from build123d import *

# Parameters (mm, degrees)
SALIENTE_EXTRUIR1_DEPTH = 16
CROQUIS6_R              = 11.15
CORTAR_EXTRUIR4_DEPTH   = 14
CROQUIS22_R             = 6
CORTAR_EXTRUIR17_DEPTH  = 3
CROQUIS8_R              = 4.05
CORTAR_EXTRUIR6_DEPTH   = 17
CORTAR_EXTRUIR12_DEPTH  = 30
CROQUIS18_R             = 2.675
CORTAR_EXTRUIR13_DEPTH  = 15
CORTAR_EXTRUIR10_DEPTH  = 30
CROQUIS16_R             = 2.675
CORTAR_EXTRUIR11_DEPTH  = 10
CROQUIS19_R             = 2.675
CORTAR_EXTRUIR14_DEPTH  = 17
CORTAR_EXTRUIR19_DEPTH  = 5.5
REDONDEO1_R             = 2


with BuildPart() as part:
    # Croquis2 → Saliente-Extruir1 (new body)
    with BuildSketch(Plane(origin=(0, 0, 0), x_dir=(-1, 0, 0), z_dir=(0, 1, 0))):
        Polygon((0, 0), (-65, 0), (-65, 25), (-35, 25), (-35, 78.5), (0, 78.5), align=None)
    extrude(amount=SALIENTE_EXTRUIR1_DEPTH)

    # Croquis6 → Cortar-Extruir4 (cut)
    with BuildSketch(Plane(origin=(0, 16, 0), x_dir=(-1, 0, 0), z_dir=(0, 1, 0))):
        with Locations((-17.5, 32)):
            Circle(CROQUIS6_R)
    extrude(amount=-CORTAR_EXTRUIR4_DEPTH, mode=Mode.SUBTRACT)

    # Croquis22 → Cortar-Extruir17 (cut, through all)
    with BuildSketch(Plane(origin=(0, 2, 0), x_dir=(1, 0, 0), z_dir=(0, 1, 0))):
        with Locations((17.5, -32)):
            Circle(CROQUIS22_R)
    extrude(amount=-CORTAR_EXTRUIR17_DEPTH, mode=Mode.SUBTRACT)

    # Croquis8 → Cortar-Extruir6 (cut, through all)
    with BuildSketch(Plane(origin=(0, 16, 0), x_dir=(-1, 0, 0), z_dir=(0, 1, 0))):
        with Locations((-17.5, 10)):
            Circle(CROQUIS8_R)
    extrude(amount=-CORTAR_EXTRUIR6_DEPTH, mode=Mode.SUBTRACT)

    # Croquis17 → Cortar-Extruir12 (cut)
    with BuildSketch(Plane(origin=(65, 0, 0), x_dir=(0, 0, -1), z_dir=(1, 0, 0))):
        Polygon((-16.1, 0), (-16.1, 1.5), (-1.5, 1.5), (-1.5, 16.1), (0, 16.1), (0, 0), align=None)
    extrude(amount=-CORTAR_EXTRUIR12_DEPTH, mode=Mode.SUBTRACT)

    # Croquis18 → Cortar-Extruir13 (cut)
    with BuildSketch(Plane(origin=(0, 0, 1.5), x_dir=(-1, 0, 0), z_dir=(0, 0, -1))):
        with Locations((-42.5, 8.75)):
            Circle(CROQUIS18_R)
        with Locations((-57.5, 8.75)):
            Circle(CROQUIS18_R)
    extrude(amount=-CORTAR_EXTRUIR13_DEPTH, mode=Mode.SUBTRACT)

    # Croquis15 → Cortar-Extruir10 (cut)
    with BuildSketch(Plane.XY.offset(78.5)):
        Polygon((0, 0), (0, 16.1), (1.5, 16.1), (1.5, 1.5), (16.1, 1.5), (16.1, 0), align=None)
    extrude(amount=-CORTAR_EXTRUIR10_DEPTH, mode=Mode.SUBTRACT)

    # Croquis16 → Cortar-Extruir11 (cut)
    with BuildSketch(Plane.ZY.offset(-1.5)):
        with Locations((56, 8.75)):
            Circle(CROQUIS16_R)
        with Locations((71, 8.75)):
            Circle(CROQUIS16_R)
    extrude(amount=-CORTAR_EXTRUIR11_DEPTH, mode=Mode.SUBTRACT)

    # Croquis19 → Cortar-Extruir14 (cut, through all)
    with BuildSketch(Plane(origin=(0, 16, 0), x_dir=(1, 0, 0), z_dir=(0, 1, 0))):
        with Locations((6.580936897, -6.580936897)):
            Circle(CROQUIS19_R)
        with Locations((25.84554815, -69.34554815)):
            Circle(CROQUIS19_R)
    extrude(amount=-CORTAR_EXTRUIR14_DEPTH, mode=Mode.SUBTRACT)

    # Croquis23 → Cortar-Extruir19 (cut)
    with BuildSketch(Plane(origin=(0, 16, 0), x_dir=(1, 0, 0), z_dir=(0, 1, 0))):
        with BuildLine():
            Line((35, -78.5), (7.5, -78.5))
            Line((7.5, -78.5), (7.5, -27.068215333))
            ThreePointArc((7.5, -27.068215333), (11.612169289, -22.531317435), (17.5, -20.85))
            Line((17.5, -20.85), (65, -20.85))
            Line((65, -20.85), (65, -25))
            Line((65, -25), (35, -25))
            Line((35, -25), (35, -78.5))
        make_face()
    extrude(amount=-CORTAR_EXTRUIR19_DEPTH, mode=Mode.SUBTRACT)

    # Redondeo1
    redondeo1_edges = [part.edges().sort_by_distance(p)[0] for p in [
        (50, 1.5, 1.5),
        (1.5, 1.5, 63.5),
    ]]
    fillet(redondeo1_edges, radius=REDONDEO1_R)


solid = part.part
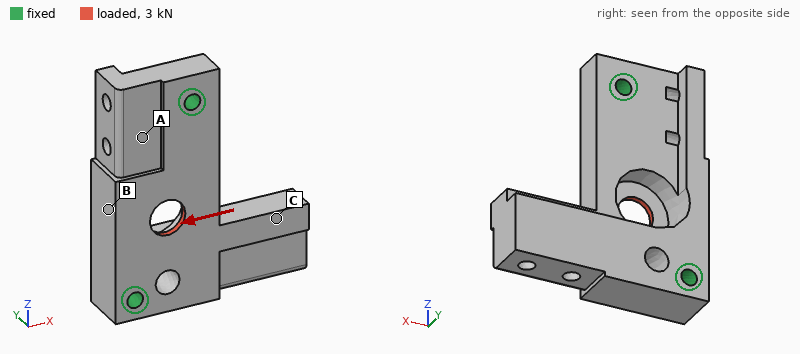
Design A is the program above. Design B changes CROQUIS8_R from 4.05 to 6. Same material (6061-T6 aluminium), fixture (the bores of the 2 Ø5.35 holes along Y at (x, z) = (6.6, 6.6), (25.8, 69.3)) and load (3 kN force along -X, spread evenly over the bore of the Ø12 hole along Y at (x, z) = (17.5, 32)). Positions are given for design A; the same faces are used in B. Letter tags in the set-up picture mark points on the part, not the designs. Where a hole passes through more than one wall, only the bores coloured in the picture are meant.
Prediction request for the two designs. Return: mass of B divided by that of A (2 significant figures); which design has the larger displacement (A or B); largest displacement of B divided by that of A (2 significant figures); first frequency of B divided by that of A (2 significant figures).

0.97
B
1.2
0.88
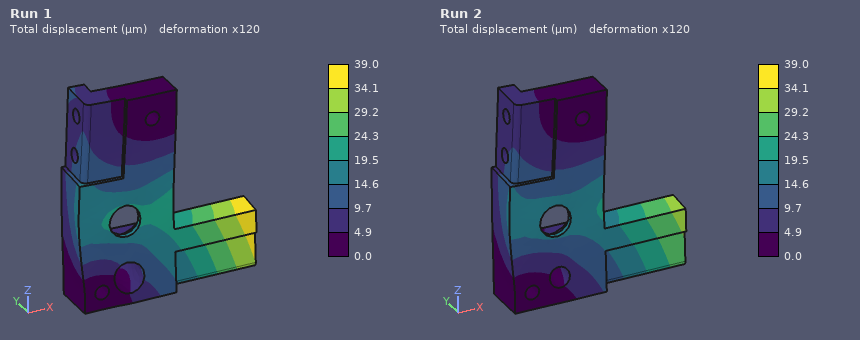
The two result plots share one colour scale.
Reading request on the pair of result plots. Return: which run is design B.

Run 1
